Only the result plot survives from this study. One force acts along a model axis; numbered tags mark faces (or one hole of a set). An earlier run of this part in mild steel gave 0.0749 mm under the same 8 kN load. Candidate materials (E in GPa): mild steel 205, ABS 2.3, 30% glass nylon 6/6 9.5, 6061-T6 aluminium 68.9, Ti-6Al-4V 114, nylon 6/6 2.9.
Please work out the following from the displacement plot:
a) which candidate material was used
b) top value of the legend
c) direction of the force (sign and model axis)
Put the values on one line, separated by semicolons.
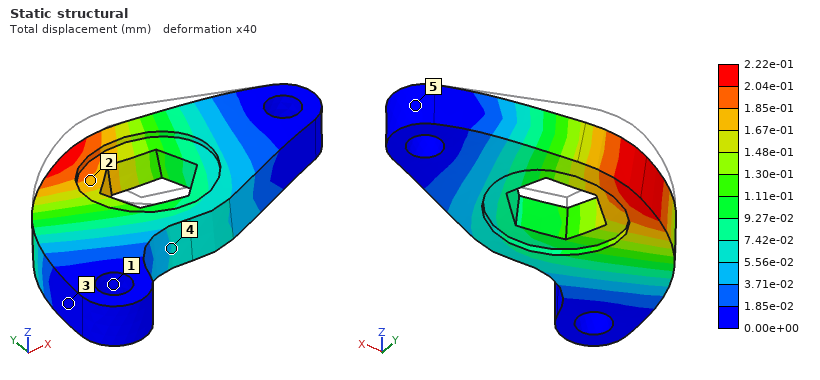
6061-T6 aluminium; 2.22e-01 mm; -Z
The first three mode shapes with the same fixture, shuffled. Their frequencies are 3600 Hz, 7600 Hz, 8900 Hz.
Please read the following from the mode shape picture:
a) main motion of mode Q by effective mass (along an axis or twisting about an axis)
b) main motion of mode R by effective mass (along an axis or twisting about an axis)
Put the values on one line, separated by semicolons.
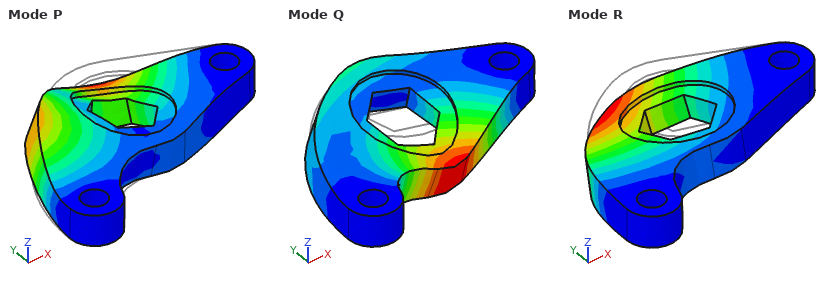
along Z; along Z
